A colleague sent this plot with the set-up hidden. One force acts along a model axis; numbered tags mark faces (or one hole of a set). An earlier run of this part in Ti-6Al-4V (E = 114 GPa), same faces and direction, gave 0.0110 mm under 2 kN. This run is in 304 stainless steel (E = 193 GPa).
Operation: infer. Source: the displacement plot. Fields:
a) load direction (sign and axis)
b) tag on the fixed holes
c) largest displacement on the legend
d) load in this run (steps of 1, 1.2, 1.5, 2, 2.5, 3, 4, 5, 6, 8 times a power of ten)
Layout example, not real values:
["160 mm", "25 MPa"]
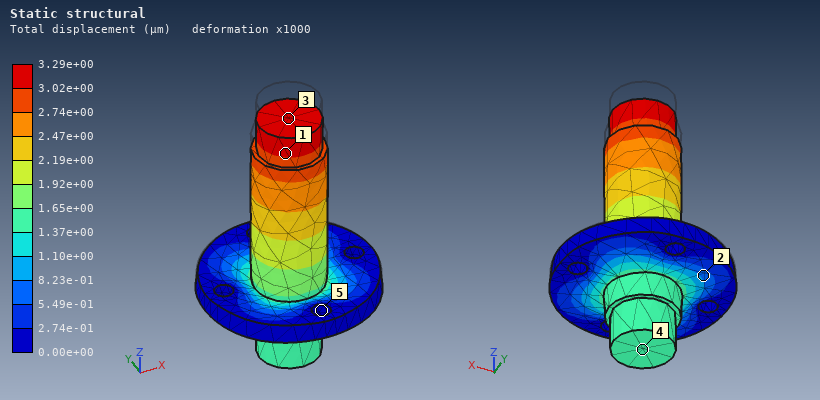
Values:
["-Z", "5", "3.29e+00 µm", "1 kN"]
